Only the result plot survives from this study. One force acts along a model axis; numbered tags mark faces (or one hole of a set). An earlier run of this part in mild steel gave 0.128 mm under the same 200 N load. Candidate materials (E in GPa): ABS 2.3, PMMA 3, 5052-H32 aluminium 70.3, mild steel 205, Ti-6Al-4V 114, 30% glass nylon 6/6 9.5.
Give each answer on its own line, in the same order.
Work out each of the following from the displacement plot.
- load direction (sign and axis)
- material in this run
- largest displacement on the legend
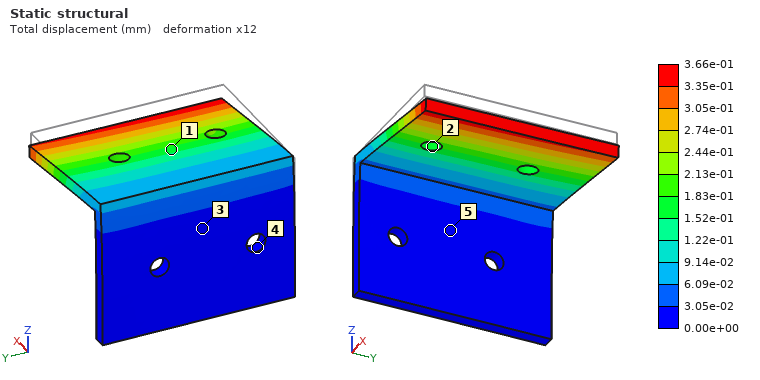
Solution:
-Z
5052-H32 aluminium
3.66e-01 mm
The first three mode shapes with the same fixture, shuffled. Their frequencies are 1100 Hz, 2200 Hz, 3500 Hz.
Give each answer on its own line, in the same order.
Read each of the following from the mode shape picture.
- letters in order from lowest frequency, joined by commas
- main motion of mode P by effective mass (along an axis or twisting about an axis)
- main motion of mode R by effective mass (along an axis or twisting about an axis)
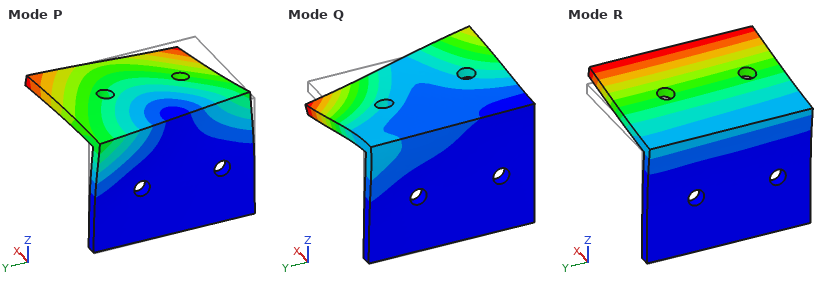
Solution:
R, P, Q
along Y
along Z
